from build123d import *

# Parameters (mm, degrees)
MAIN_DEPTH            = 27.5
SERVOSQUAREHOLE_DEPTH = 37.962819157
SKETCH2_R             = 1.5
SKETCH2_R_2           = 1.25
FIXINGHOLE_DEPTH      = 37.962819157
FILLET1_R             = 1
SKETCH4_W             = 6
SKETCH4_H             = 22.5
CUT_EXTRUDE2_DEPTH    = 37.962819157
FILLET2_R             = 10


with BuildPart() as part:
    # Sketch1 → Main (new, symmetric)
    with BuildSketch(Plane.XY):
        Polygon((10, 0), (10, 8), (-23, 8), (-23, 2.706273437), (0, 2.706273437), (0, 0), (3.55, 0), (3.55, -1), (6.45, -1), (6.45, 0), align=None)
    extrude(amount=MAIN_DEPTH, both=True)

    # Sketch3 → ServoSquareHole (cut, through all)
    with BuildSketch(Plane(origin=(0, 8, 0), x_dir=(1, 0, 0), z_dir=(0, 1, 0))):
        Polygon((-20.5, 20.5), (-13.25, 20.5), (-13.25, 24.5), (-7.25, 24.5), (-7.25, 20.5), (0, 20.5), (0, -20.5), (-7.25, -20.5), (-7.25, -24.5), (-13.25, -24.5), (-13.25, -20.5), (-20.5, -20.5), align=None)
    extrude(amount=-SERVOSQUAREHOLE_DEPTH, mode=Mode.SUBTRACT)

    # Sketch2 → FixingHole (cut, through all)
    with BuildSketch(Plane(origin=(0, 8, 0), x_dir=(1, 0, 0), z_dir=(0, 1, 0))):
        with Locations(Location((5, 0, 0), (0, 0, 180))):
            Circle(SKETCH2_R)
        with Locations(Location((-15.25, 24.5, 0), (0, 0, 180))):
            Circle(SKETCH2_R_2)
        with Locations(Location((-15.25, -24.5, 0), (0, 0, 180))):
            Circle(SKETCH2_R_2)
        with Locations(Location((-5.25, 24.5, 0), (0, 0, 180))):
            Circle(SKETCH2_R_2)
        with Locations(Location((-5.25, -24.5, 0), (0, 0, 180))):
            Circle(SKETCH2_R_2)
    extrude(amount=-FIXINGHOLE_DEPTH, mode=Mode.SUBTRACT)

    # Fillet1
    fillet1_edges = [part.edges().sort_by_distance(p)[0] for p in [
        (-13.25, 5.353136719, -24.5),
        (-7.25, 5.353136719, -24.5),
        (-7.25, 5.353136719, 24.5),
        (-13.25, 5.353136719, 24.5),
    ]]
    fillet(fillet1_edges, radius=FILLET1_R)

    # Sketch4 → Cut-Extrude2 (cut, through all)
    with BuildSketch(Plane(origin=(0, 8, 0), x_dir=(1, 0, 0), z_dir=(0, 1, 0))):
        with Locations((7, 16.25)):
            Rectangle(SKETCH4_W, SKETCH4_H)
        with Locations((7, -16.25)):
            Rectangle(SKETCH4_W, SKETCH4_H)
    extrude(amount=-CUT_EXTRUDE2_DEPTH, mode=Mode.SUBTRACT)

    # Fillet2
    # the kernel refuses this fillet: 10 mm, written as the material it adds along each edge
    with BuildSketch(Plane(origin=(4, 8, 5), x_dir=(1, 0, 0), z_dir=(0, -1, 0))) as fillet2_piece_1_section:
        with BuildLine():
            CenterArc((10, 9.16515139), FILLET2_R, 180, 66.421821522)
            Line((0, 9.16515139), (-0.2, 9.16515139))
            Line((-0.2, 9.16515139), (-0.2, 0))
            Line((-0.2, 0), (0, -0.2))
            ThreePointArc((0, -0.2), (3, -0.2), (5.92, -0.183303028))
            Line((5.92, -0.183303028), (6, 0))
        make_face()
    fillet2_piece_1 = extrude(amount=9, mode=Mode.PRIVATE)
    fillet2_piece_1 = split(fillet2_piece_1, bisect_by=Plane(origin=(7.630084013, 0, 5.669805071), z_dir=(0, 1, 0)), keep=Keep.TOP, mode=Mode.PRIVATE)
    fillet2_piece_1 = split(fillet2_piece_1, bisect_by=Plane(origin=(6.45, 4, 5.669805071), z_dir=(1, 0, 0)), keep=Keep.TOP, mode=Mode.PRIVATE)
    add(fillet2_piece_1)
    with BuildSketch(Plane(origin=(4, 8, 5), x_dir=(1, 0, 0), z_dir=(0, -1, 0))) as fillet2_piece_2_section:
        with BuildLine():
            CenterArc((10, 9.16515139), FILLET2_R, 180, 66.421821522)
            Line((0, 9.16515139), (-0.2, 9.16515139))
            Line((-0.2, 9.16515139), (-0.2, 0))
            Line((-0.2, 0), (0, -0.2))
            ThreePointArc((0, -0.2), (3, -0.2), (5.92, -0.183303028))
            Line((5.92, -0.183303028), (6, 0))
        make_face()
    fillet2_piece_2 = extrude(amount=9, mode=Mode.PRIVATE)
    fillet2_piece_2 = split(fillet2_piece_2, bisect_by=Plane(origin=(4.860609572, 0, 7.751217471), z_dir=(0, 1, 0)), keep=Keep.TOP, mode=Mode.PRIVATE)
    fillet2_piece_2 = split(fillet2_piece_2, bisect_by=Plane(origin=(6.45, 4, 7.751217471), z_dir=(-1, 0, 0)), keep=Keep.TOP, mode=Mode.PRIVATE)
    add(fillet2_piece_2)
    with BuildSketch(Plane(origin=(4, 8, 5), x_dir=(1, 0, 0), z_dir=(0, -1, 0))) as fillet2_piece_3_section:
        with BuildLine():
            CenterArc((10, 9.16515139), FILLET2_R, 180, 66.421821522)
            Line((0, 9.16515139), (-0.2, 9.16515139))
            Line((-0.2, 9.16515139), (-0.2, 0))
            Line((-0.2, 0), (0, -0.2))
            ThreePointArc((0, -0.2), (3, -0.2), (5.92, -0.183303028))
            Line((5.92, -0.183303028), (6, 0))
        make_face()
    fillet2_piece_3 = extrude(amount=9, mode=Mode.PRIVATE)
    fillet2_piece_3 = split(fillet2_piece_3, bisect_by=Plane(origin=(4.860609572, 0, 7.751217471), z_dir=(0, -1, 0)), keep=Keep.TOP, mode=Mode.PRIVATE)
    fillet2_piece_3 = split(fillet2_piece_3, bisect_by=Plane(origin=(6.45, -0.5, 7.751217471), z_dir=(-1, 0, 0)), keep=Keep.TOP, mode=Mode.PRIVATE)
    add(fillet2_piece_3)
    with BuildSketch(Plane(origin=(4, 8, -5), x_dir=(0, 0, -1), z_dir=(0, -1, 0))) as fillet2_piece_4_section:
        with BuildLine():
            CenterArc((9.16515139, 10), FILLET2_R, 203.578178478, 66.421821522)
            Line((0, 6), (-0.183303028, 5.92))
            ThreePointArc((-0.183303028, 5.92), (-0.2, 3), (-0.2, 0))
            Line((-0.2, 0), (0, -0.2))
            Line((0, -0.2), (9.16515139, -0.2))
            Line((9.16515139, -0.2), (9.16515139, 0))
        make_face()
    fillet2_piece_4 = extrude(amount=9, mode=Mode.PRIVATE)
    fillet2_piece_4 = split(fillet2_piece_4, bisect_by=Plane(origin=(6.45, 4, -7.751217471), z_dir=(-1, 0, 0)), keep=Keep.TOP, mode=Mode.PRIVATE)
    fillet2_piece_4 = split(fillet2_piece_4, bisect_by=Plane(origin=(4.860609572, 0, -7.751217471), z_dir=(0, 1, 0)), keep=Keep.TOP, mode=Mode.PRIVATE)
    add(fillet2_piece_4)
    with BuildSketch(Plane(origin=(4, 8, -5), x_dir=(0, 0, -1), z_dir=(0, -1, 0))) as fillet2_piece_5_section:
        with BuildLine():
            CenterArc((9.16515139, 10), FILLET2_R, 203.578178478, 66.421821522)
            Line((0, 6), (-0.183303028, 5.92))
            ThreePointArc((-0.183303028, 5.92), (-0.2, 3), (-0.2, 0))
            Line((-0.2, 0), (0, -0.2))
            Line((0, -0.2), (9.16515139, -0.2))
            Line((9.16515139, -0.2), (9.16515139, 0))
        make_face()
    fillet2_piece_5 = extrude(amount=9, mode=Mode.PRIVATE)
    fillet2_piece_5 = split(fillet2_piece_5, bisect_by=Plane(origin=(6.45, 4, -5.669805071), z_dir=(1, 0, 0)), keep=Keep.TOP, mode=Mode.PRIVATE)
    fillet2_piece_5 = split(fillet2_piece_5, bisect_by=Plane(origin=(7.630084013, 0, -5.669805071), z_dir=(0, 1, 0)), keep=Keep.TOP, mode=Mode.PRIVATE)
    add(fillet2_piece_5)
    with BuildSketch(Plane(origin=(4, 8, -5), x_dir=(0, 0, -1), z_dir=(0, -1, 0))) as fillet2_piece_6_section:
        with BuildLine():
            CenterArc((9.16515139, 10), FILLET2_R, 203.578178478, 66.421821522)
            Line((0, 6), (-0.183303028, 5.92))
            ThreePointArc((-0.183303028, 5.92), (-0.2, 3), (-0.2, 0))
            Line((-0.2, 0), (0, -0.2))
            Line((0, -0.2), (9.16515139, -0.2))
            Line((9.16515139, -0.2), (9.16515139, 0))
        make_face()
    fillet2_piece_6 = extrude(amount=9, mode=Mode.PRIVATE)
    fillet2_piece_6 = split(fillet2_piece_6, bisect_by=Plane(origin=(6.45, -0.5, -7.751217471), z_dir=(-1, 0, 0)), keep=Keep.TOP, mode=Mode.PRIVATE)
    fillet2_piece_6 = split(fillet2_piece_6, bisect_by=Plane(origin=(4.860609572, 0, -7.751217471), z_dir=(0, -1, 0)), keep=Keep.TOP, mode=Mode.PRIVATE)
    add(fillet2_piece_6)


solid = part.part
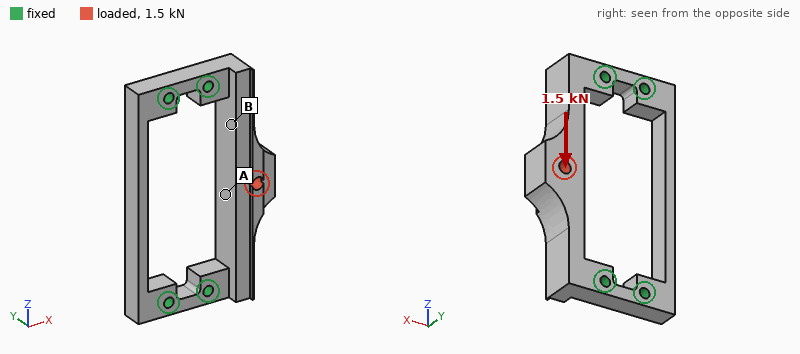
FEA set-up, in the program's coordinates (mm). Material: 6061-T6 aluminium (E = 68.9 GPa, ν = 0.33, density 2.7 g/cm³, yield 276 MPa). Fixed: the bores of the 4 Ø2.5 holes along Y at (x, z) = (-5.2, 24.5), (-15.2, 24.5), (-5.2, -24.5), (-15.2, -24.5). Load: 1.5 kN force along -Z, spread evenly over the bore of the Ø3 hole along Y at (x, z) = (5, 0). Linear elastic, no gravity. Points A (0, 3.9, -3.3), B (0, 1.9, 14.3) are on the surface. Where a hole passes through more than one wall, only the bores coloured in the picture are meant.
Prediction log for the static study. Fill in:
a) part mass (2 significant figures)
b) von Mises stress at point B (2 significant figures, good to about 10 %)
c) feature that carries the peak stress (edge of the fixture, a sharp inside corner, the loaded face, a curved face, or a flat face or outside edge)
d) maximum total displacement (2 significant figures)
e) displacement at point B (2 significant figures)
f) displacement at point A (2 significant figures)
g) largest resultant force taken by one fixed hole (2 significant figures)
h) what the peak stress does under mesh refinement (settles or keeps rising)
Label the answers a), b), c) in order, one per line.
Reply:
a) 12 g
b) 29 MPa
c) edge of the fixture
d) 21 µm
e) 19 µm
f) 21 µm
g) 800 N
h) keeps rising
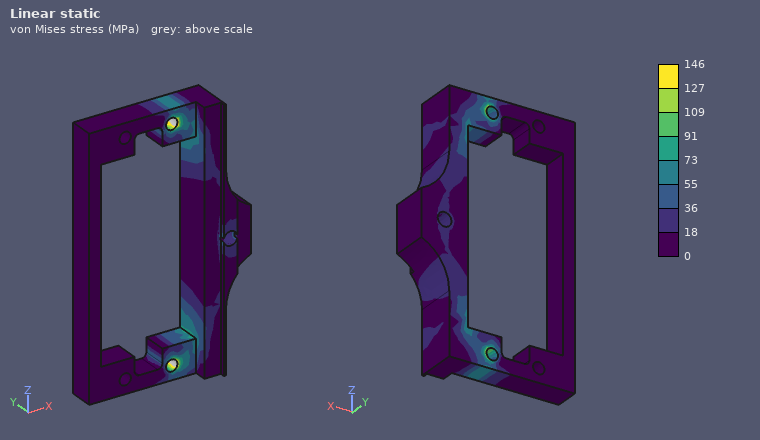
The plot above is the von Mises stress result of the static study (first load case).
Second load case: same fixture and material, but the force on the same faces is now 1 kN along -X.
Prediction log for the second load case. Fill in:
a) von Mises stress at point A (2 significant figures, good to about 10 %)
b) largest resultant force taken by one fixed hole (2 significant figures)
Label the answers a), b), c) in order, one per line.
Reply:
a) 42 MPa
b) 770 N
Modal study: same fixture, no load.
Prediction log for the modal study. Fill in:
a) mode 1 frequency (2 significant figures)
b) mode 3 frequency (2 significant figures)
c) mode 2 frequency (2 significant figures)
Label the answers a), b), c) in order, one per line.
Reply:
a) 6600 Hz
b) 10 kHz
c) 6800 Hz
